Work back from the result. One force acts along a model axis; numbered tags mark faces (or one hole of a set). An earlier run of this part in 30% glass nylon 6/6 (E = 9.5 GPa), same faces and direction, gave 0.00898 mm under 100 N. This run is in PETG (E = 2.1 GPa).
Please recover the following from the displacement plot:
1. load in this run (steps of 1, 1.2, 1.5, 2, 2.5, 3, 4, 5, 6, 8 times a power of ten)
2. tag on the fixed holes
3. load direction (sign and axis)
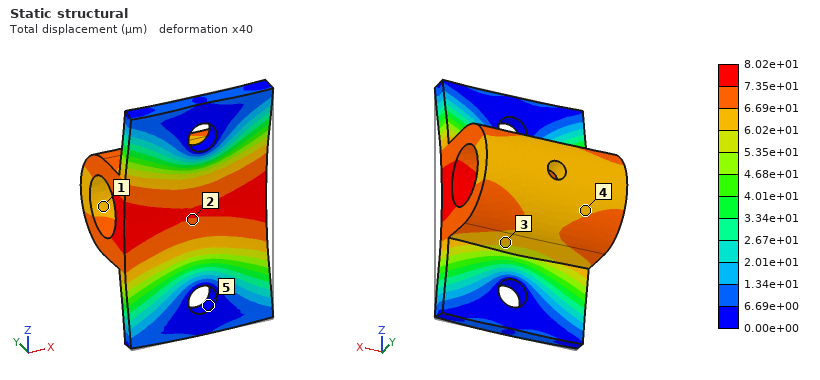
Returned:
200 N
5
+Y
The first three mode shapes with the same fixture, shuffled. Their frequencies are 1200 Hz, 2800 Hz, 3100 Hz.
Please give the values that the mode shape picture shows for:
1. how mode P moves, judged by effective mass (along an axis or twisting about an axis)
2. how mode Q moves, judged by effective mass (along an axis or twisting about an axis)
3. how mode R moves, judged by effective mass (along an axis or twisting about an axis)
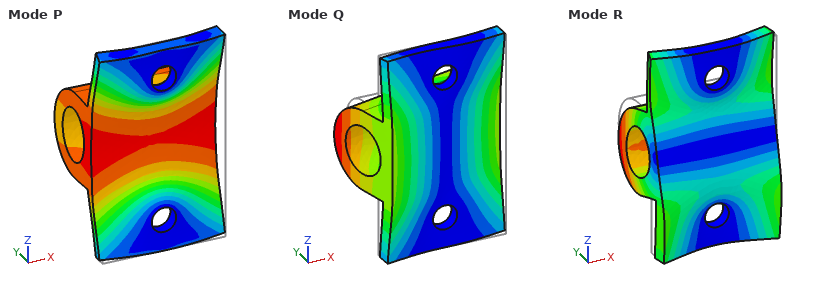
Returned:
along Y
along X
along Z
